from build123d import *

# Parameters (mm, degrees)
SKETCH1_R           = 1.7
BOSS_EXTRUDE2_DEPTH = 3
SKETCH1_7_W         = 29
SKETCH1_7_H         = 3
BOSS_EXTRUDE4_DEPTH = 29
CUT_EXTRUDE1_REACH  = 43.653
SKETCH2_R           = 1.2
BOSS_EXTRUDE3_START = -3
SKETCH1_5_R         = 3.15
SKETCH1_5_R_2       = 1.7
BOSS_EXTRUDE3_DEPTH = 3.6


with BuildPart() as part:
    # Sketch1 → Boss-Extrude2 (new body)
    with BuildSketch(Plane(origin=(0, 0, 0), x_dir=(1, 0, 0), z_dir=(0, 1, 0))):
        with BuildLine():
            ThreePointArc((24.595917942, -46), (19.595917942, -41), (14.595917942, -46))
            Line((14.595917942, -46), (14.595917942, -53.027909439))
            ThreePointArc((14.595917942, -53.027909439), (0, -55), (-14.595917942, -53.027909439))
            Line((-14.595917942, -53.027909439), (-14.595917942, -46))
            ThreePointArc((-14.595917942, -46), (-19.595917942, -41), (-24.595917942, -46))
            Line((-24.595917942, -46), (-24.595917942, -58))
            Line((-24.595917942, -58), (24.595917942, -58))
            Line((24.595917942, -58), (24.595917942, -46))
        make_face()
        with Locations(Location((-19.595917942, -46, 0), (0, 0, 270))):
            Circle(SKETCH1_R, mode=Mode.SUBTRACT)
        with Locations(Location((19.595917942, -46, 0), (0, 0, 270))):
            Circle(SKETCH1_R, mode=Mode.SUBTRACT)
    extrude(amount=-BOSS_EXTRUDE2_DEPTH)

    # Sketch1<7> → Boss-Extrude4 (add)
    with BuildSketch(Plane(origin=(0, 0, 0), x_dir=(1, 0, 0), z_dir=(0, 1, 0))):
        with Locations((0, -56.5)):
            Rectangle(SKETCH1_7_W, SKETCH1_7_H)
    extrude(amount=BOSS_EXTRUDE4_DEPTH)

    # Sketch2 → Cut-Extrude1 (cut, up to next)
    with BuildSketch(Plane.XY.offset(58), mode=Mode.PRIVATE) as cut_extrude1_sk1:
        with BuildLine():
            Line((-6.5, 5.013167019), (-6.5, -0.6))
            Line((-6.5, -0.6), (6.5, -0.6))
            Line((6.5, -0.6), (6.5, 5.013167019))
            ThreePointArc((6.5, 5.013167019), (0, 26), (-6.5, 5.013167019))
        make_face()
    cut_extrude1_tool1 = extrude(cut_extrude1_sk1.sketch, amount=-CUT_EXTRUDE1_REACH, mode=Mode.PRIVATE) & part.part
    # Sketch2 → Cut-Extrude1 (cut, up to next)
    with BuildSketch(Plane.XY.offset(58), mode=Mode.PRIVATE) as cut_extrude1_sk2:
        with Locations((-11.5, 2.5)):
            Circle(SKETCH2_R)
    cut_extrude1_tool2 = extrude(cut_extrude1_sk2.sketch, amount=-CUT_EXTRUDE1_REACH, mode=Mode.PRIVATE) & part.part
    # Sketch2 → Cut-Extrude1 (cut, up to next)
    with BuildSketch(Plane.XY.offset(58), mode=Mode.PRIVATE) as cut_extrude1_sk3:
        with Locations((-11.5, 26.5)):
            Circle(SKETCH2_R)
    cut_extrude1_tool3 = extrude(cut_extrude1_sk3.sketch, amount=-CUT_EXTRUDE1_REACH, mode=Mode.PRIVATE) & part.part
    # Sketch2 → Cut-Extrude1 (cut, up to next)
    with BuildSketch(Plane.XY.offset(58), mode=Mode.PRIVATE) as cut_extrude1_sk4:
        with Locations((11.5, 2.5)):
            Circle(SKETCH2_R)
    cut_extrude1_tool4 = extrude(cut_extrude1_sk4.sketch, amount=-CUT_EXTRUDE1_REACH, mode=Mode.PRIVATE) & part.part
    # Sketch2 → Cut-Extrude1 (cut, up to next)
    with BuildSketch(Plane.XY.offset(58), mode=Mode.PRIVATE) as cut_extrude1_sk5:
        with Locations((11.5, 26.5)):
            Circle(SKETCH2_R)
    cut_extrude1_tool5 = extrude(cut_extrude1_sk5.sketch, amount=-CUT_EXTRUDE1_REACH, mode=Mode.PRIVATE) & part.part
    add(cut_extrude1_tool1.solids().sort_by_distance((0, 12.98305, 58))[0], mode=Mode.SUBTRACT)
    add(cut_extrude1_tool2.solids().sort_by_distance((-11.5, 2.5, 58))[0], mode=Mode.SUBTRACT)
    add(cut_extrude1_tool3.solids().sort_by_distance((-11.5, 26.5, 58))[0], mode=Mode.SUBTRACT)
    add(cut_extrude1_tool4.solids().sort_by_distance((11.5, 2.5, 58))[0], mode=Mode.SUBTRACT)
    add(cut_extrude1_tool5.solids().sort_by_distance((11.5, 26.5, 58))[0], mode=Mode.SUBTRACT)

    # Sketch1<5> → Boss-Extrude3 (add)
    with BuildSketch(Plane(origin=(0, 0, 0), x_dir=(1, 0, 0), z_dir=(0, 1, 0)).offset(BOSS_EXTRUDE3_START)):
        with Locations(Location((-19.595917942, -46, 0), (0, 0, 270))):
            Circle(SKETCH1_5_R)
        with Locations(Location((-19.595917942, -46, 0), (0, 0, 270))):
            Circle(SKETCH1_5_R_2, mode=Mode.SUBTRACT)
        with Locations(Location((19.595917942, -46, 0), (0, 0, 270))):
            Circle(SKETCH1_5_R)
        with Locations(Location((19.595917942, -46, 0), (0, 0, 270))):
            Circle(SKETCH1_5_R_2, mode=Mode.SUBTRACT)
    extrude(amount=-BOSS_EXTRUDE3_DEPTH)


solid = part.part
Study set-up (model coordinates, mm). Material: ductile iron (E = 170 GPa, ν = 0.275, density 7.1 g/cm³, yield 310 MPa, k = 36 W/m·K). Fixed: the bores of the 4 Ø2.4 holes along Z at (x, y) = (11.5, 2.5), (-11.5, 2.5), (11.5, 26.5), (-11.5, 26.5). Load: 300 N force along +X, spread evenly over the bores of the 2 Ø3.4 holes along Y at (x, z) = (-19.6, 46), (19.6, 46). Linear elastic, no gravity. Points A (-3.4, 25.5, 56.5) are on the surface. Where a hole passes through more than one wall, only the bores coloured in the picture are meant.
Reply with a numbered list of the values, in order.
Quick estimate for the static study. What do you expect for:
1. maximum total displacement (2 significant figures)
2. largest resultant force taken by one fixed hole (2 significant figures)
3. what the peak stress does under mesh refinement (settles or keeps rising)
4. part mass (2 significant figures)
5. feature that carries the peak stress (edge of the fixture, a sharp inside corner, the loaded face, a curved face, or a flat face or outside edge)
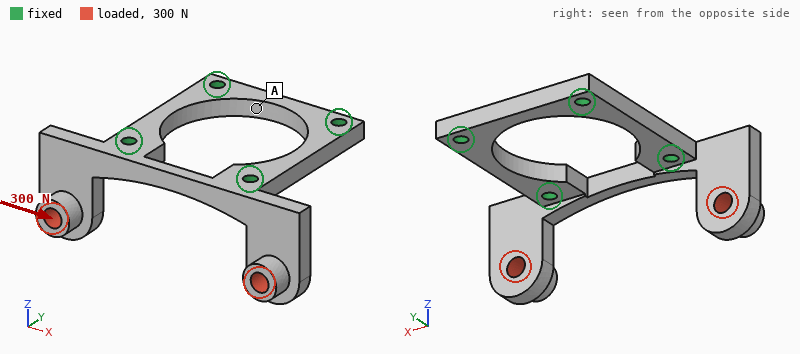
1. 48 µm
2. 160 N
3. keeps rising
4. 17 g
5. edge of the fixture
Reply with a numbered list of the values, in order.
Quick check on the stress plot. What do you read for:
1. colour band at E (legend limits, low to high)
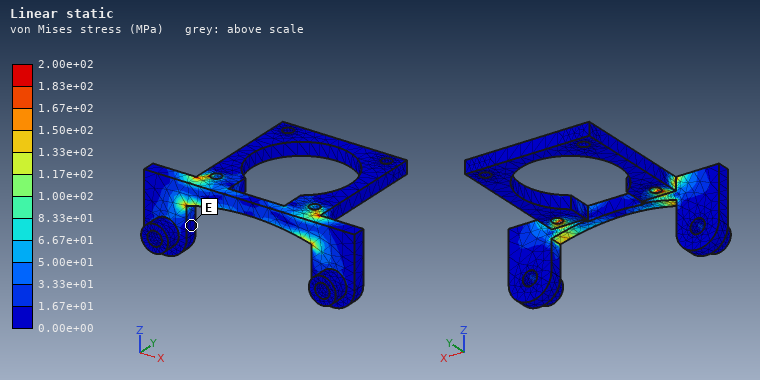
1. 0.00e+00 to 1.67e+01 MPa
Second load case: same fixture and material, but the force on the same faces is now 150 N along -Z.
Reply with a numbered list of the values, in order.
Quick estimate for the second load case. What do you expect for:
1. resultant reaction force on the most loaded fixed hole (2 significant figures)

1. 75 N
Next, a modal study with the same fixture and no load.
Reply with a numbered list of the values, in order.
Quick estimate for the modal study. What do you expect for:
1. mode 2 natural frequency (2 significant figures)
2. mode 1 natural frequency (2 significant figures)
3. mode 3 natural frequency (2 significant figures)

1. 4500 Hz
2. 4500 Hz
3. 5600 Hz
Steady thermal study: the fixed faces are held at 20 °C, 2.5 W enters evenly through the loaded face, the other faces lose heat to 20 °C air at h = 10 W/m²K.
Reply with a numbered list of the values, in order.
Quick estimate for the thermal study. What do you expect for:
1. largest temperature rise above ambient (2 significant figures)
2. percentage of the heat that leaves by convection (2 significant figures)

1. 26 K
2. 8.7 %
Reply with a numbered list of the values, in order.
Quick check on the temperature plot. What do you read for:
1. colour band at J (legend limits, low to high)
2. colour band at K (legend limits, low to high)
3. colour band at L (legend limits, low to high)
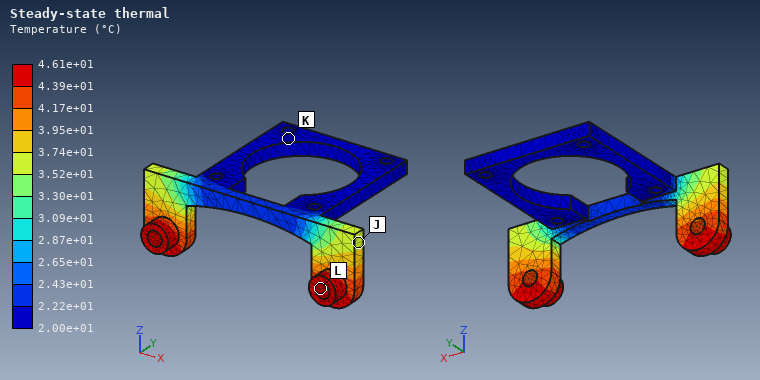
1. 3.52e+01 to 3.74e+01 °C
2. 2.00e+01 to 2.22e+01 °C
3. 4.39e+01 to 4.61e+01 °C
